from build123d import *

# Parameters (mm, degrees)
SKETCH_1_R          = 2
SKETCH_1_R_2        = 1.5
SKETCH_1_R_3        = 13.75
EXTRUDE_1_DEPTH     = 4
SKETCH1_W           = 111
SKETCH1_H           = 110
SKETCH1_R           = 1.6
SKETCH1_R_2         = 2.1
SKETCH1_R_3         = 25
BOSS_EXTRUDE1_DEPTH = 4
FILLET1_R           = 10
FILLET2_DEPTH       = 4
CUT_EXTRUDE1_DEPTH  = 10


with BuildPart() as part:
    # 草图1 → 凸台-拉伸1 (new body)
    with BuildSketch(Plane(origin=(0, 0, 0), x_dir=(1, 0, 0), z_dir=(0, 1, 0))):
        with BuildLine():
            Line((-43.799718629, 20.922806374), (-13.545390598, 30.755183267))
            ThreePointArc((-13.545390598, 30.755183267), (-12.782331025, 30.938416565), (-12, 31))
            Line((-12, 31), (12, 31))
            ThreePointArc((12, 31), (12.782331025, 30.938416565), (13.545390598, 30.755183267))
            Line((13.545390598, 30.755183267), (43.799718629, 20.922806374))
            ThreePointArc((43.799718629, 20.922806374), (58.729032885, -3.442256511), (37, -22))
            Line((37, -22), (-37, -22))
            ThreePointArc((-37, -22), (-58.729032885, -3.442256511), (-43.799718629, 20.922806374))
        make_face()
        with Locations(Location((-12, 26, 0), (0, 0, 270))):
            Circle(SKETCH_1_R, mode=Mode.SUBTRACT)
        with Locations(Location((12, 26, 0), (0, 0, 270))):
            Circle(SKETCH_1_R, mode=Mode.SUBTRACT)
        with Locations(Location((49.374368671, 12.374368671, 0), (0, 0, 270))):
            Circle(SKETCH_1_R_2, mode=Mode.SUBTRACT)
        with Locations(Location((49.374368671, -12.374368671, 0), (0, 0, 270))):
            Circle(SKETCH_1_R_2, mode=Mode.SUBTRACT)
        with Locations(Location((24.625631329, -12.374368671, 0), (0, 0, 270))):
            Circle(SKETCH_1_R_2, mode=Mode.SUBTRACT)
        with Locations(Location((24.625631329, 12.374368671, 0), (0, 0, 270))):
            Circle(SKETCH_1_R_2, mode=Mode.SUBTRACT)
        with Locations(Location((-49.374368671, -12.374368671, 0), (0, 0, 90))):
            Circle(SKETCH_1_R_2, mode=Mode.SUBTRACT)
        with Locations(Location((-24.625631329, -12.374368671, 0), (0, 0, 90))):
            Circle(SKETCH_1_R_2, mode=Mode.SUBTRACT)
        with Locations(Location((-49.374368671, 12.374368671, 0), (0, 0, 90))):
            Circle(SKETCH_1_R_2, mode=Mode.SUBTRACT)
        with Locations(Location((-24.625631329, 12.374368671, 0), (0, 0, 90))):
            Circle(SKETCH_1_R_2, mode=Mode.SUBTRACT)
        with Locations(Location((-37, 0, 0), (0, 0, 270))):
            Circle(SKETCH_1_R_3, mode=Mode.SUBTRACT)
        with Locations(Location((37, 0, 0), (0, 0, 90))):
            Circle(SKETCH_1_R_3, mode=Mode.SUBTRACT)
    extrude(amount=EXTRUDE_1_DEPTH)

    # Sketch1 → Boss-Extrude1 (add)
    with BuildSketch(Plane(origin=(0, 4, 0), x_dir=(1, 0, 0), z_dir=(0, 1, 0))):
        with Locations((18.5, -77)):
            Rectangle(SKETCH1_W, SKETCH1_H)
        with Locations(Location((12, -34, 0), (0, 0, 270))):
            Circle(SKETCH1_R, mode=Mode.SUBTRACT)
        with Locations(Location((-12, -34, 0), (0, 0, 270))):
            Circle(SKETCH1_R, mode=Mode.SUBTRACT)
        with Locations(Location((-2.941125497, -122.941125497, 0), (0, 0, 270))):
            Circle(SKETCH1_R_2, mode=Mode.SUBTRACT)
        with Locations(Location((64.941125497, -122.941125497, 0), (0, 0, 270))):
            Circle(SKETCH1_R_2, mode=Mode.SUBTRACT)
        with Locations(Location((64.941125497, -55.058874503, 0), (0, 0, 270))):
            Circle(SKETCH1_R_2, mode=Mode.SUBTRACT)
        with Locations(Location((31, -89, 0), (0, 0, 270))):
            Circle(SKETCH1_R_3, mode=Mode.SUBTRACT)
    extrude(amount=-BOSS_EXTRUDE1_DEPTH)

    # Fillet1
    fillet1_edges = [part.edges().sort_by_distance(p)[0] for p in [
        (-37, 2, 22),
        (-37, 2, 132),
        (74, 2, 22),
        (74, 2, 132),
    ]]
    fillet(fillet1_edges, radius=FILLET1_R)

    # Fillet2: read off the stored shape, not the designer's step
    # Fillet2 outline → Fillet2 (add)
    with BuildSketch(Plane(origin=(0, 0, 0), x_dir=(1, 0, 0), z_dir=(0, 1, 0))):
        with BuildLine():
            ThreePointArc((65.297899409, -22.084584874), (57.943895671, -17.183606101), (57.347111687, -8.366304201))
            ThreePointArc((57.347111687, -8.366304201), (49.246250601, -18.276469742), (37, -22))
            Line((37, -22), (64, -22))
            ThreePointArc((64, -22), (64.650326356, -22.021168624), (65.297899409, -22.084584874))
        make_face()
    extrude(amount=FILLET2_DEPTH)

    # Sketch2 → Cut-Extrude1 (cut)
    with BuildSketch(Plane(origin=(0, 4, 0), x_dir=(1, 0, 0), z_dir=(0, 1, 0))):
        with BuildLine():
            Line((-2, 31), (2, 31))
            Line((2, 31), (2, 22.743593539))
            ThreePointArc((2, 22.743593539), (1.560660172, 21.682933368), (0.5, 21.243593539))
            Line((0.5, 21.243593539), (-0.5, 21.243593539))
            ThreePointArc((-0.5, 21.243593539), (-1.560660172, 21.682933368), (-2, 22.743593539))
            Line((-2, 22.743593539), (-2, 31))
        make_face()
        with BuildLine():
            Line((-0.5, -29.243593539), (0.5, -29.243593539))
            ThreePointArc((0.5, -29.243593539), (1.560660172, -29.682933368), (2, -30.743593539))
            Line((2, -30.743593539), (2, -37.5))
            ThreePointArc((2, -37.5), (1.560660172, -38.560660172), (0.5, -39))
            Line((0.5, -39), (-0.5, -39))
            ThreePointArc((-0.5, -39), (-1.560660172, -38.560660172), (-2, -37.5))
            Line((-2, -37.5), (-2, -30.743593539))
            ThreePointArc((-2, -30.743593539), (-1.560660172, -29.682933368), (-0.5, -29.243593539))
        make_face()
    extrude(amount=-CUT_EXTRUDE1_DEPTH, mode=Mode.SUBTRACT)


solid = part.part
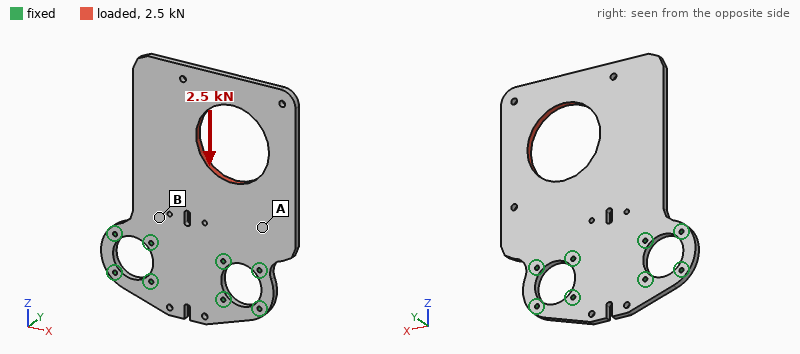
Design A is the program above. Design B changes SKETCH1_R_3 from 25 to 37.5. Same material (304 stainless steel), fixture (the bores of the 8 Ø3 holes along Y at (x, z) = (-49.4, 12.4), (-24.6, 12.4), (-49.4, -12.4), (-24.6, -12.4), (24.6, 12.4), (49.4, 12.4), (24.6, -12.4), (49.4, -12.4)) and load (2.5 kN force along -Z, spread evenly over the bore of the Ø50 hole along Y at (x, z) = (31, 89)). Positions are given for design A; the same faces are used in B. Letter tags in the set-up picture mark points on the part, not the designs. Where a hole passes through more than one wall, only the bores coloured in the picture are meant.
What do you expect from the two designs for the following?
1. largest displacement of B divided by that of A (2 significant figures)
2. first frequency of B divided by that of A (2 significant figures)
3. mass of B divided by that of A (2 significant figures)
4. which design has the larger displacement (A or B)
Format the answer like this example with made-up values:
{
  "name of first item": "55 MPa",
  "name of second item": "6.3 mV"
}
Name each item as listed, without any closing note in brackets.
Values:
{
  "largest displacement of B divided by that of A": "4.2",
  "first frequency of B divided by that of A": "1.1",
  "mass of B divided by that of A": "0.83",
  "which design has the larger displacement": "B"
}
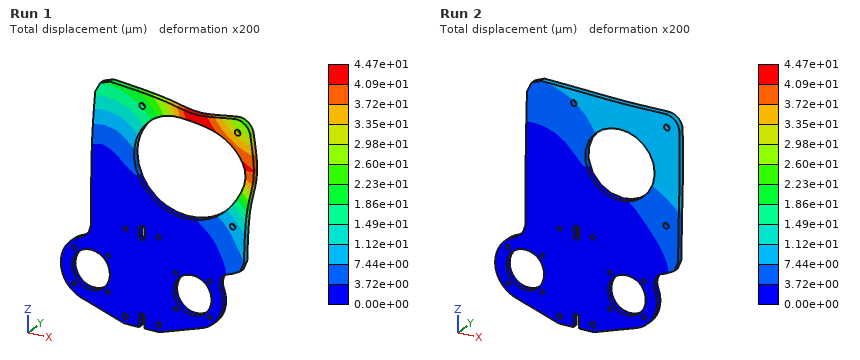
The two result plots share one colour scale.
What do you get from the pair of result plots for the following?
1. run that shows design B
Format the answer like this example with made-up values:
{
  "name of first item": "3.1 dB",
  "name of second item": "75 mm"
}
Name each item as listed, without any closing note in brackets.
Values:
{
  "run that shows design B": "Run 1"
}
